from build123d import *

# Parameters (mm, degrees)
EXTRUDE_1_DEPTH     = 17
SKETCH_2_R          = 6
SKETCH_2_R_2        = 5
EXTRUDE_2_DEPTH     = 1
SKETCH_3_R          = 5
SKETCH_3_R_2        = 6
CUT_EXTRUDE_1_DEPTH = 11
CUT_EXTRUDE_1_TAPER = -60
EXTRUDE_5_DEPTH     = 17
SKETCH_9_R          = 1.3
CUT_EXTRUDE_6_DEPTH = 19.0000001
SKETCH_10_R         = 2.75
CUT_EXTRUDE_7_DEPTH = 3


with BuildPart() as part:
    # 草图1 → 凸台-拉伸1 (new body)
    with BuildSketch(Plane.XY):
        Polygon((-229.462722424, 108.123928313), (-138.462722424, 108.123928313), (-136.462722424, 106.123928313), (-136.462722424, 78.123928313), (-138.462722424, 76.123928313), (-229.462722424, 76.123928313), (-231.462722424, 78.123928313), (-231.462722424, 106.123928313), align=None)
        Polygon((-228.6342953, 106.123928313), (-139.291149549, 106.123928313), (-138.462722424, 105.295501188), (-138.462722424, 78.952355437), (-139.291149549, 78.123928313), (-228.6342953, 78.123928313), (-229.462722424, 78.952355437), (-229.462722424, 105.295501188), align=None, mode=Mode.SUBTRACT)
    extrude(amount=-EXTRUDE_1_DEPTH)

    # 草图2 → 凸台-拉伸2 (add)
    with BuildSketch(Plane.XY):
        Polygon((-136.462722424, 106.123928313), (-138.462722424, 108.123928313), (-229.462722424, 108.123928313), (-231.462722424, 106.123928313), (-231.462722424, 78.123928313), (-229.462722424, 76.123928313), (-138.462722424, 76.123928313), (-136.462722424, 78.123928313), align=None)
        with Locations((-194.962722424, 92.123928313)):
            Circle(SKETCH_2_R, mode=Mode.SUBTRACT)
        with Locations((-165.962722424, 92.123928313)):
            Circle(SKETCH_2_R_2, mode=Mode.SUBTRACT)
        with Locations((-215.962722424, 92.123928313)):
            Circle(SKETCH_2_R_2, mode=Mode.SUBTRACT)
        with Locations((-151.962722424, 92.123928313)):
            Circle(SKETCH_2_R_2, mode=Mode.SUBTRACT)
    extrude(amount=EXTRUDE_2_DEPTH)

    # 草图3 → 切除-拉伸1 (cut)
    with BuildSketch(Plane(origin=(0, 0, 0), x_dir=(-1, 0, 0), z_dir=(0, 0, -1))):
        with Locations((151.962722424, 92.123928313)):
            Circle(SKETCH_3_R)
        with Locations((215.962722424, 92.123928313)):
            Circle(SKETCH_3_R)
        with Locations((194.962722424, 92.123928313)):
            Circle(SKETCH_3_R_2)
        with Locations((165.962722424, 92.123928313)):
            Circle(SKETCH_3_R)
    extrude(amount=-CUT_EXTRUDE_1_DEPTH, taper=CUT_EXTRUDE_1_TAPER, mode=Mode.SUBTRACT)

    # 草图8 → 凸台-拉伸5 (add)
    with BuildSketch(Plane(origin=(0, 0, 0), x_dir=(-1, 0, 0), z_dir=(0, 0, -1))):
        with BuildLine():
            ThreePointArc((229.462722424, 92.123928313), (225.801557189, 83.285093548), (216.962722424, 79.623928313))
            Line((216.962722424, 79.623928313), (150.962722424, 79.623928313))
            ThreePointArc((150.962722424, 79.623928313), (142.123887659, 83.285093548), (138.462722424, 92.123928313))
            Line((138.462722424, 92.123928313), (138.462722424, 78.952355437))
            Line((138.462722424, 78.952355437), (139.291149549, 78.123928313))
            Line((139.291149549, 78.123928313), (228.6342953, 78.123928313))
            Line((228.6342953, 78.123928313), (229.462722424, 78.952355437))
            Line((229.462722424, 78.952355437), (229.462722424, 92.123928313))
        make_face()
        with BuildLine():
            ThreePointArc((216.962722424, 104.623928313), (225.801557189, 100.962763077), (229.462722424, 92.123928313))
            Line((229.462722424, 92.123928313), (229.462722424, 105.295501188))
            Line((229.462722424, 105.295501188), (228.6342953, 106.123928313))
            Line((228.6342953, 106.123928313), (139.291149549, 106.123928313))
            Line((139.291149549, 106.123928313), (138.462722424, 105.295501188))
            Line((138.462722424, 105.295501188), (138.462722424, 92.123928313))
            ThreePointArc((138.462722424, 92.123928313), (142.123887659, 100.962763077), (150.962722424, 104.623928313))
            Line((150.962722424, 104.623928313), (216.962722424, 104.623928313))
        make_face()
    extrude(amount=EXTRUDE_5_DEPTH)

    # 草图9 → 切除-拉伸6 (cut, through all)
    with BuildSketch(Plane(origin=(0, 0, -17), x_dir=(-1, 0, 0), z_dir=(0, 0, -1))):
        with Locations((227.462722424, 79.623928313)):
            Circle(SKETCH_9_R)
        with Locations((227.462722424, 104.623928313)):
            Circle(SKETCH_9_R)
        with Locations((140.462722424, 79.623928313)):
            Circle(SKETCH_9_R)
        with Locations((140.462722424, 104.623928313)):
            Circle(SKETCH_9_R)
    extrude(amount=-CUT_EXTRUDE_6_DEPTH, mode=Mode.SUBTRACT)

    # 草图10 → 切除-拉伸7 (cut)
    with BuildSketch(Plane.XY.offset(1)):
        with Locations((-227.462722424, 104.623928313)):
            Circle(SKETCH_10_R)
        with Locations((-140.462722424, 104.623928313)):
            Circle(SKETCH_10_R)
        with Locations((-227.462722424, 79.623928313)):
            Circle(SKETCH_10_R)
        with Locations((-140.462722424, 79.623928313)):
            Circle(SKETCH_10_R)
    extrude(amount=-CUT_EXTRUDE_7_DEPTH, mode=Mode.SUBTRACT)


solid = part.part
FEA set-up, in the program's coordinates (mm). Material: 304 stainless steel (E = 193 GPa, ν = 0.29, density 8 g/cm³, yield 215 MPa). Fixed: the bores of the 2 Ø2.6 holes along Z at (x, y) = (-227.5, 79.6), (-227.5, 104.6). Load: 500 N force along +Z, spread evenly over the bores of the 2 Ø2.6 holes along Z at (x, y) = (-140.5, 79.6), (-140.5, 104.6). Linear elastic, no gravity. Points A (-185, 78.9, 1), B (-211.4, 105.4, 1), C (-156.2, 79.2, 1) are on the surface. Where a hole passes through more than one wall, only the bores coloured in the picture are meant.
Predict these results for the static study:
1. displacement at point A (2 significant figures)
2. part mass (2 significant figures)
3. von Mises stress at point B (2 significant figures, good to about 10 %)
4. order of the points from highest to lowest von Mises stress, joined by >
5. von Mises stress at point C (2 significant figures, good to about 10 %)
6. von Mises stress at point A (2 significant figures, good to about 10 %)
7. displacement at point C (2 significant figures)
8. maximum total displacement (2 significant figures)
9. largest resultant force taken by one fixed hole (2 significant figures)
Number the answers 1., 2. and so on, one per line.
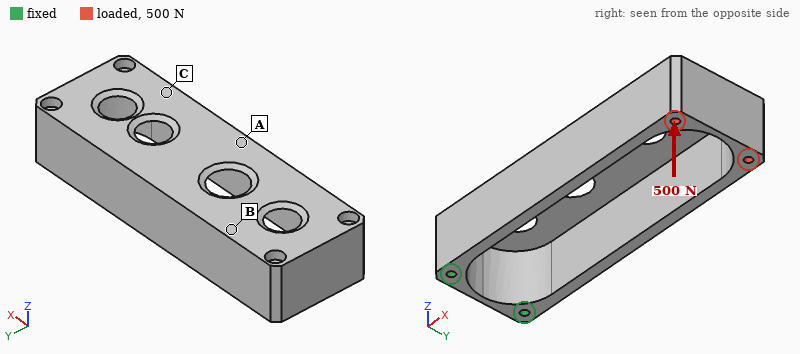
1. 0.048 mm
2. 140 g
3. 68 MPa
4. B > A > C
5. 16 MPa
6. 43 MPa
7. 0.11 mm
8. 0.16 mm
9. 270 N
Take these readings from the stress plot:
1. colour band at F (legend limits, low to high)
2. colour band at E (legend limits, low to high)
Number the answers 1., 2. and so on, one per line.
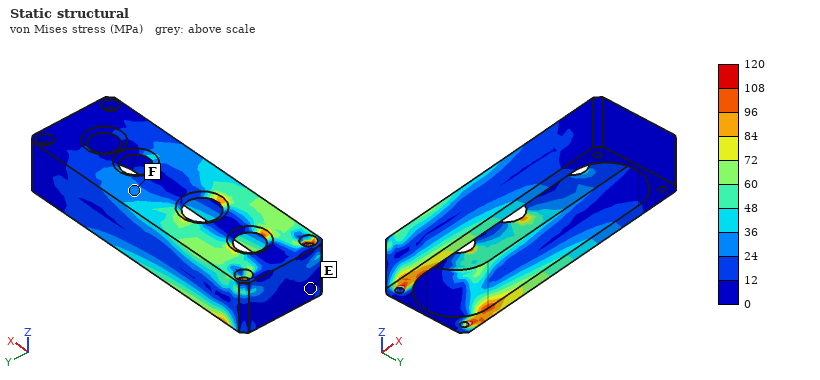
1. 24 to 36 MPa
2. 0 to 12 MPa
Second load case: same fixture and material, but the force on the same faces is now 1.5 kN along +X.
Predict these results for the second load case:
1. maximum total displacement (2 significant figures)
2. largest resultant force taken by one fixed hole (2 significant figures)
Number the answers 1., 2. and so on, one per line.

1. 20 µm
2. 750 N
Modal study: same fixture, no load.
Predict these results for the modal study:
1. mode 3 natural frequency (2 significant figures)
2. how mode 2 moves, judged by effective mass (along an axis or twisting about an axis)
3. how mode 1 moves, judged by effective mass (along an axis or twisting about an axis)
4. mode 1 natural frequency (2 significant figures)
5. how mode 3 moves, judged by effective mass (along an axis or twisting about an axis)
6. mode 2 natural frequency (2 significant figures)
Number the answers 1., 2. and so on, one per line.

1. 3500 Hz
2. along Z
3. along Y
4. 1200 Hz
5. along Y
6. 1400 Hz
